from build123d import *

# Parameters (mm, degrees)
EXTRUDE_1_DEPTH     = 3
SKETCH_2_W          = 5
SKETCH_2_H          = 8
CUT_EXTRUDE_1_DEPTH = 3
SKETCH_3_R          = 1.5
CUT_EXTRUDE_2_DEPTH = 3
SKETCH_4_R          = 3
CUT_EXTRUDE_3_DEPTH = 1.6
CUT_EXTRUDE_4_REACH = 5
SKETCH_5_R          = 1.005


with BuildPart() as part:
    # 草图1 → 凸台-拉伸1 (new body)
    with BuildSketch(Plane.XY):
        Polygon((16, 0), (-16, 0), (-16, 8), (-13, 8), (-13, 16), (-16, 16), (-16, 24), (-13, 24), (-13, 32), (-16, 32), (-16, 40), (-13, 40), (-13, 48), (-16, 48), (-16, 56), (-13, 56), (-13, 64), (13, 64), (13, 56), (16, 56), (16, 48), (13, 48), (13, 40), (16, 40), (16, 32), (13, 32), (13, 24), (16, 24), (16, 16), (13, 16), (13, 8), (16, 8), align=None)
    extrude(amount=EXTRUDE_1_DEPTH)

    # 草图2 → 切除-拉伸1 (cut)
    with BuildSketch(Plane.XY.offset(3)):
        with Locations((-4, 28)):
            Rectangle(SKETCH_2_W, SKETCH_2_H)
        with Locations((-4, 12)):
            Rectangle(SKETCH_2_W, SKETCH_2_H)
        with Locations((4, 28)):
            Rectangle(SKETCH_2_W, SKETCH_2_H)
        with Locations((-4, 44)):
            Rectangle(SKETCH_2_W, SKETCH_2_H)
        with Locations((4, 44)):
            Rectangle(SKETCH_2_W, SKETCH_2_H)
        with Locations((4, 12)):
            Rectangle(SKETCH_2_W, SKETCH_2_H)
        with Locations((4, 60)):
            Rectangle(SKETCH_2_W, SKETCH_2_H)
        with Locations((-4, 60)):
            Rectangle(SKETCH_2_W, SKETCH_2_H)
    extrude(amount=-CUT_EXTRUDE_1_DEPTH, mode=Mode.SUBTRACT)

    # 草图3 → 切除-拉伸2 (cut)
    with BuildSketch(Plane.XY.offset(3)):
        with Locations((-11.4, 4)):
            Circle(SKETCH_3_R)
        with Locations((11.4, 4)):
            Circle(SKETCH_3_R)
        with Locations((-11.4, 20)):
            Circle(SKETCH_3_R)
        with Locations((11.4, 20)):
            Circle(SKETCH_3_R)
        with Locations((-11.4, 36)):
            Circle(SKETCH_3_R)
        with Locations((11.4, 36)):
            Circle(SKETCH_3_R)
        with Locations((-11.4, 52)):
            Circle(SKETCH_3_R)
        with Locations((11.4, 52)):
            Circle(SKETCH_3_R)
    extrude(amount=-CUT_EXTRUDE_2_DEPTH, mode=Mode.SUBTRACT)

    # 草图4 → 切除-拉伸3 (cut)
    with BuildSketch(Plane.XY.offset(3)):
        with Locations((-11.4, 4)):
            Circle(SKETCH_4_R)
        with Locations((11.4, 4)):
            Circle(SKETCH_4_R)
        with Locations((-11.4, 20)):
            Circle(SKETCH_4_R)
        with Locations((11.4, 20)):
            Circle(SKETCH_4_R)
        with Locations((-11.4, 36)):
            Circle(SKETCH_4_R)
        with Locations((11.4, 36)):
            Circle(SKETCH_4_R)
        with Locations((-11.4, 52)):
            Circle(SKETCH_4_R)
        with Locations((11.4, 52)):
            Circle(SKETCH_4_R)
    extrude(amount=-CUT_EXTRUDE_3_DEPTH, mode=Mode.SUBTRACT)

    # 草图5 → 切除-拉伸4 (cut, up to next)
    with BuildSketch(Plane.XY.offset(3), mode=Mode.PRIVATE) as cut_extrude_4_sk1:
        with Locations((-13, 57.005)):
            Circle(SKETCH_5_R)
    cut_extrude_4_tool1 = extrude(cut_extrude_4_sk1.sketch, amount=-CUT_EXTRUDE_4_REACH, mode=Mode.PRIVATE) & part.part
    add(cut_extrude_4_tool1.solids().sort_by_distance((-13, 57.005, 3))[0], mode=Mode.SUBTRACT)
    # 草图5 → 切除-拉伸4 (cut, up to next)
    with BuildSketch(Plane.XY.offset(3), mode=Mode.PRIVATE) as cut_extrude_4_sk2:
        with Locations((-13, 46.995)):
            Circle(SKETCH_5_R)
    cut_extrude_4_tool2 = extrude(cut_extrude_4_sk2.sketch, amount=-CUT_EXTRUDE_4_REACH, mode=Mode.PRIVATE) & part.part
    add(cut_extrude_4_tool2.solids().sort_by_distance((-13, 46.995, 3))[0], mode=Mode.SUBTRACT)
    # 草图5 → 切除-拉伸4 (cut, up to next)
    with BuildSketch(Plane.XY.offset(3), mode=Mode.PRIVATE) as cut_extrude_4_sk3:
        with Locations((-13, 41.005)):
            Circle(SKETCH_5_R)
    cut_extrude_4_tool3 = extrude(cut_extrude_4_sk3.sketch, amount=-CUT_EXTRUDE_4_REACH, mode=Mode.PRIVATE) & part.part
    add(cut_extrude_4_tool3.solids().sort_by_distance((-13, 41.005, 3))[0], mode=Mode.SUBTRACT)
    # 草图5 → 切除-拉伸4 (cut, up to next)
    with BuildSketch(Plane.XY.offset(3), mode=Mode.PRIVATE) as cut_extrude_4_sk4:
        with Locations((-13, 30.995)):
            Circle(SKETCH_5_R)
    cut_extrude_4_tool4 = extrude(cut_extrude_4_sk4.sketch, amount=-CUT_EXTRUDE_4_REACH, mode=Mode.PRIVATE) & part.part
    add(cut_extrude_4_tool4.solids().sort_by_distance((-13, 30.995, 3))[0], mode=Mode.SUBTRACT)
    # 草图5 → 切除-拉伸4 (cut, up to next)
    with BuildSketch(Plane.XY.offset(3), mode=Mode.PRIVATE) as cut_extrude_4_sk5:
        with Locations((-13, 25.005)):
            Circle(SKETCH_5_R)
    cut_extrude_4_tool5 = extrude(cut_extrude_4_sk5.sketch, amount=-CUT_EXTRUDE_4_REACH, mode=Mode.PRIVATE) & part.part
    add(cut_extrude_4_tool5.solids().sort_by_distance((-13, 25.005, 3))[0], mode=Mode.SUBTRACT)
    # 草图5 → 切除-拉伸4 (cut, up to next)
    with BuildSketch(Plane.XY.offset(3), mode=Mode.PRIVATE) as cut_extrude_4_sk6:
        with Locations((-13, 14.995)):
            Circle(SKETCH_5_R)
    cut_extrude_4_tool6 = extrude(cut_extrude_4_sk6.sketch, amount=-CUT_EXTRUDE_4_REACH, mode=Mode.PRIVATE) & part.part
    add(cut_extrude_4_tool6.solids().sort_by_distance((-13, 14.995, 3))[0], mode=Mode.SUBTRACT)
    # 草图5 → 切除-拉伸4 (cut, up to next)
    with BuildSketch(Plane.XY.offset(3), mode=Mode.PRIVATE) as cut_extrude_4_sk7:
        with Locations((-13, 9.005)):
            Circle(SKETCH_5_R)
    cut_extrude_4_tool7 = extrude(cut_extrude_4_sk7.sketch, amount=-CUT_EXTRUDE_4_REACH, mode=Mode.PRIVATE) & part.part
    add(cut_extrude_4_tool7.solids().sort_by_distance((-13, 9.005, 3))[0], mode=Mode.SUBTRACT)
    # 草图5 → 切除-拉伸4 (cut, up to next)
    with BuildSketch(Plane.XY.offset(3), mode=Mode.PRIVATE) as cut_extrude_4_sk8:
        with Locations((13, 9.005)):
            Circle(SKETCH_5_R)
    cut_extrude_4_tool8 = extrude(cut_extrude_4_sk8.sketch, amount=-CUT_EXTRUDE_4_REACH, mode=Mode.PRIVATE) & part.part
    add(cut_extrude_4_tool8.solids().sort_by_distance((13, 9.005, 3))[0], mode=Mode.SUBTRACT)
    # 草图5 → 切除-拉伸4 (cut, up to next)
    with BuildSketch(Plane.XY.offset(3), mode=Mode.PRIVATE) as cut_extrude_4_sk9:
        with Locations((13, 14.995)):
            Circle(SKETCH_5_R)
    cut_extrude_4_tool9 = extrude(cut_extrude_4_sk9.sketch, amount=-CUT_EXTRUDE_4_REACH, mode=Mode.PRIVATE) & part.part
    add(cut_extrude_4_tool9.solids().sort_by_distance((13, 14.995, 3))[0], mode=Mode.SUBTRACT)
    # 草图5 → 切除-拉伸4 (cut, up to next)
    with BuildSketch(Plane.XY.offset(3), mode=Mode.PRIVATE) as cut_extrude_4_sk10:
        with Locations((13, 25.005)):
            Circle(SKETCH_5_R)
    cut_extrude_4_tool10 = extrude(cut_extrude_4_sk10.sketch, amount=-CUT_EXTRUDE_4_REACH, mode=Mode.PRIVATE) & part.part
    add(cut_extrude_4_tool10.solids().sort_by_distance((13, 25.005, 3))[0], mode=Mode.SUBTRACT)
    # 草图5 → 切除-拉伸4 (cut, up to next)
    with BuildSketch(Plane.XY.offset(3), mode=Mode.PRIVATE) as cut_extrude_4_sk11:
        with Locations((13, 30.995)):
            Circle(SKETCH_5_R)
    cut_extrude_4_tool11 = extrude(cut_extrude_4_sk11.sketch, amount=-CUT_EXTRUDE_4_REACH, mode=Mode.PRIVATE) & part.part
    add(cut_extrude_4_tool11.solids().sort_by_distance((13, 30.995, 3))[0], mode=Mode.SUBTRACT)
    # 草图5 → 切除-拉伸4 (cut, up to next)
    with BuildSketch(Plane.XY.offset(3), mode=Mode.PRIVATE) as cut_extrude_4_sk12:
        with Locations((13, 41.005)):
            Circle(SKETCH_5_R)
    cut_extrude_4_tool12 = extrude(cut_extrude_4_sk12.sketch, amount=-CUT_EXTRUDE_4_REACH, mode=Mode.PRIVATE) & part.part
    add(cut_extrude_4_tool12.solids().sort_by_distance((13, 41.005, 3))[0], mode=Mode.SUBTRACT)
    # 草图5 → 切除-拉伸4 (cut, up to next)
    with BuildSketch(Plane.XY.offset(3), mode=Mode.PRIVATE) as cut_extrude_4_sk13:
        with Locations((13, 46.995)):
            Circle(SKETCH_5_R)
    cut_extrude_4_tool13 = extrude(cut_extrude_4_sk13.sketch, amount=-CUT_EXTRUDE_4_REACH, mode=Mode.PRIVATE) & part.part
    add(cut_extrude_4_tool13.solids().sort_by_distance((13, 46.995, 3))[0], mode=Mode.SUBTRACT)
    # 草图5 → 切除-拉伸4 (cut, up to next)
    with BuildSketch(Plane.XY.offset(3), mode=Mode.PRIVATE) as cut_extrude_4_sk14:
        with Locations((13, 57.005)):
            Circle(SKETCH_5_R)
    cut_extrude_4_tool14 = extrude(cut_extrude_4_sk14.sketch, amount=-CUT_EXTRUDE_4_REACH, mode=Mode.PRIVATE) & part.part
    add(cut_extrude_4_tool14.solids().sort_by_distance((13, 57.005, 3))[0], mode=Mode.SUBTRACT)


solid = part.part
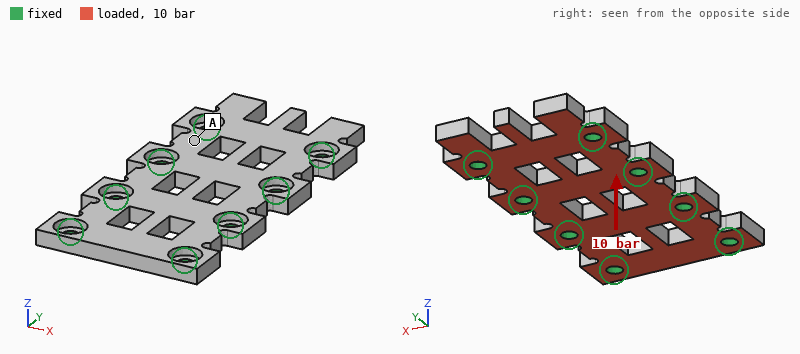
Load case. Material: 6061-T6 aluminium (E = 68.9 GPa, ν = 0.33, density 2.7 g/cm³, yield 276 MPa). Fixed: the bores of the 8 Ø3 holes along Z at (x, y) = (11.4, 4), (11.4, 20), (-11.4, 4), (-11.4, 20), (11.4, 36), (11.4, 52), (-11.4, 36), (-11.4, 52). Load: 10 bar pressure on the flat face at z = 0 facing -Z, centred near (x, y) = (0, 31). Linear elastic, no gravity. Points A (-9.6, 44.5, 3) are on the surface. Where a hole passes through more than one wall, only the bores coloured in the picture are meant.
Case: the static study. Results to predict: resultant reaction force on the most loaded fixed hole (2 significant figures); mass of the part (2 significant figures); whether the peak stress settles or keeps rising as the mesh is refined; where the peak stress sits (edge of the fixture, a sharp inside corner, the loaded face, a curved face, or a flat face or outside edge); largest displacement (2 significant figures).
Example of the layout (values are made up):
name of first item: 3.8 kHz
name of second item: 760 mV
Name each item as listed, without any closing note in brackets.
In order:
resultant reaction force on the most loaded fixed hole: 260 N
mass of the part: 11 g
whether the peak stress settles or keeps rising as the mesh is refined: keeps rising
where the peak stress sits: edge of the fixture
largest displacement: 36 µm
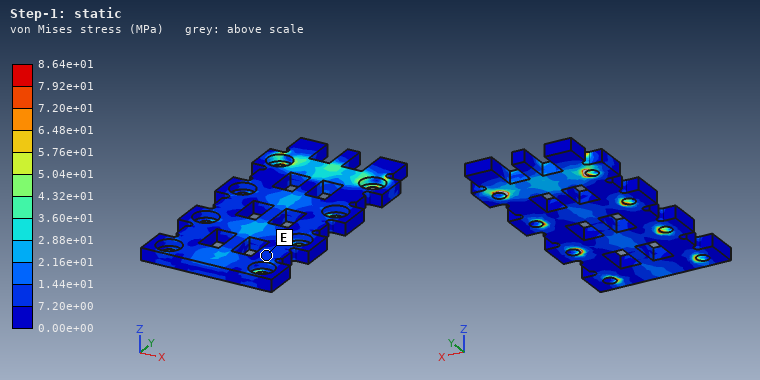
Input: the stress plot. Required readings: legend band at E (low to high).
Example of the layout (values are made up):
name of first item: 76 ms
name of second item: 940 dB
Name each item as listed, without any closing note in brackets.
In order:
legend band at E: 7.20e+00 to 1.44e+01 MPa
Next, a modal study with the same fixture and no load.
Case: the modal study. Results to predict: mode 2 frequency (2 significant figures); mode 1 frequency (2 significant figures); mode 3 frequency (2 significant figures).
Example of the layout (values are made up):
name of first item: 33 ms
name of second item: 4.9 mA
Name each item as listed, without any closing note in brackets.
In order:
mode 2 frequency: 14 kHz
mode 1 frequency: 12 kHz
mode 3 frequency: 17 kHz
